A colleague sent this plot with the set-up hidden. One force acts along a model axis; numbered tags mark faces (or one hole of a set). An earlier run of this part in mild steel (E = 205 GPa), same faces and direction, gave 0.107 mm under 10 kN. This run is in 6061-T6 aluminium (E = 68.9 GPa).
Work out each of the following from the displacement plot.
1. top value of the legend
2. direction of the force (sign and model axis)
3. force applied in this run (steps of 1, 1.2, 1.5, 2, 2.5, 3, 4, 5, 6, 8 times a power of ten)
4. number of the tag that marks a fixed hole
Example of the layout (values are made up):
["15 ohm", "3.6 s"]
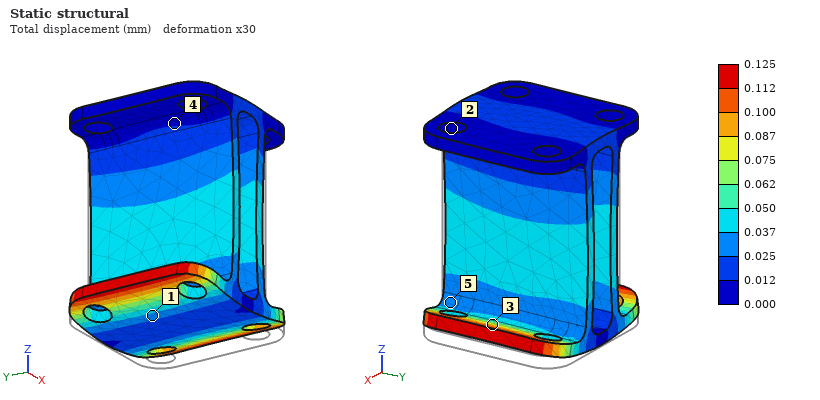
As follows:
["0.125 mm", "+Z", "4 kN", "2"]
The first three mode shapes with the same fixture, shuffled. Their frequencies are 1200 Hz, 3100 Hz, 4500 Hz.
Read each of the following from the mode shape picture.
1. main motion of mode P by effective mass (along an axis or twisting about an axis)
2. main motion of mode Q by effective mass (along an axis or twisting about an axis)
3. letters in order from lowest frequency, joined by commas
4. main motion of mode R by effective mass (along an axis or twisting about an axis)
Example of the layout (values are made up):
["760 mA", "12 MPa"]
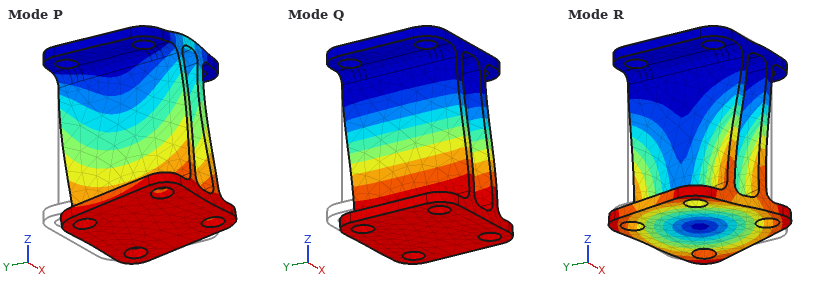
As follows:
["along Y", "along X", "Q, R, P", "twisting about Z"]
